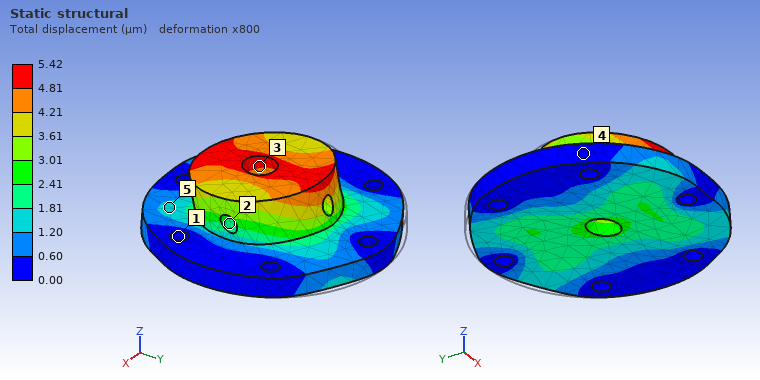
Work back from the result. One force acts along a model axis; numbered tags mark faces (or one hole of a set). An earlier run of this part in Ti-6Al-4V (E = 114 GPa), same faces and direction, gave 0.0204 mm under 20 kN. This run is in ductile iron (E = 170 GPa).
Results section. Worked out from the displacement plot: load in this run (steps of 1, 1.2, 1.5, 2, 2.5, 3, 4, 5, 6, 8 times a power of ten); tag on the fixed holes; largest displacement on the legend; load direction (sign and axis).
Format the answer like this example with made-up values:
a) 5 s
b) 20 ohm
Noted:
a) 8 kN
b) 1
c) 5.42 µm
d) -Y
